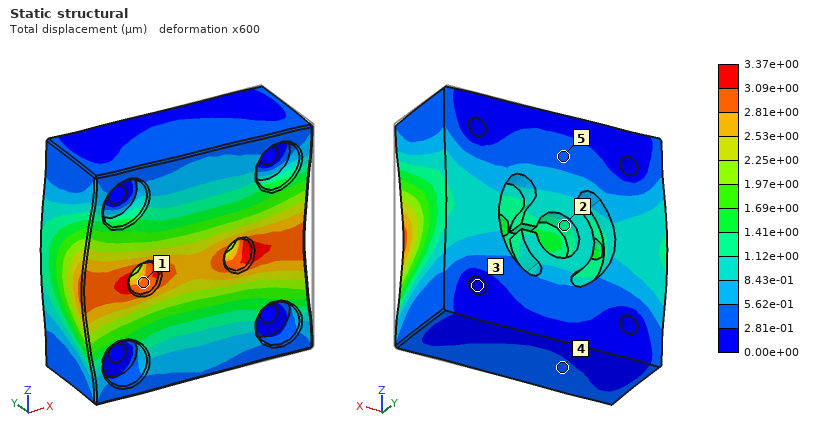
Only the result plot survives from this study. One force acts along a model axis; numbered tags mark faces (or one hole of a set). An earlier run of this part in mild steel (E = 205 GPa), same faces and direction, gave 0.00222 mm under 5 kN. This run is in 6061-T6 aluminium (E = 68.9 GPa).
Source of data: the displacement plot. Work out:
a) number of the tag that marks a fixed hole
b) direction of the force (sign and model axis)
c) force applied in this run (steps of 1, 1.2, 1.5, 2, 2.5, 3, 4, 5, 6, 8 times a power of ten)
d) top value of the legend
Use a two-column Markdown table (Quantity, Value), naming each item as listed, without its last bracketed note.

| Quantity | Value |
|---|---|
| number of the tag that marks a fixed hole | 3 |
| direction of the force | -X |
| force applied in this run | 2.5 kN |
| top value of the legend | 3.37e+00 µm |
